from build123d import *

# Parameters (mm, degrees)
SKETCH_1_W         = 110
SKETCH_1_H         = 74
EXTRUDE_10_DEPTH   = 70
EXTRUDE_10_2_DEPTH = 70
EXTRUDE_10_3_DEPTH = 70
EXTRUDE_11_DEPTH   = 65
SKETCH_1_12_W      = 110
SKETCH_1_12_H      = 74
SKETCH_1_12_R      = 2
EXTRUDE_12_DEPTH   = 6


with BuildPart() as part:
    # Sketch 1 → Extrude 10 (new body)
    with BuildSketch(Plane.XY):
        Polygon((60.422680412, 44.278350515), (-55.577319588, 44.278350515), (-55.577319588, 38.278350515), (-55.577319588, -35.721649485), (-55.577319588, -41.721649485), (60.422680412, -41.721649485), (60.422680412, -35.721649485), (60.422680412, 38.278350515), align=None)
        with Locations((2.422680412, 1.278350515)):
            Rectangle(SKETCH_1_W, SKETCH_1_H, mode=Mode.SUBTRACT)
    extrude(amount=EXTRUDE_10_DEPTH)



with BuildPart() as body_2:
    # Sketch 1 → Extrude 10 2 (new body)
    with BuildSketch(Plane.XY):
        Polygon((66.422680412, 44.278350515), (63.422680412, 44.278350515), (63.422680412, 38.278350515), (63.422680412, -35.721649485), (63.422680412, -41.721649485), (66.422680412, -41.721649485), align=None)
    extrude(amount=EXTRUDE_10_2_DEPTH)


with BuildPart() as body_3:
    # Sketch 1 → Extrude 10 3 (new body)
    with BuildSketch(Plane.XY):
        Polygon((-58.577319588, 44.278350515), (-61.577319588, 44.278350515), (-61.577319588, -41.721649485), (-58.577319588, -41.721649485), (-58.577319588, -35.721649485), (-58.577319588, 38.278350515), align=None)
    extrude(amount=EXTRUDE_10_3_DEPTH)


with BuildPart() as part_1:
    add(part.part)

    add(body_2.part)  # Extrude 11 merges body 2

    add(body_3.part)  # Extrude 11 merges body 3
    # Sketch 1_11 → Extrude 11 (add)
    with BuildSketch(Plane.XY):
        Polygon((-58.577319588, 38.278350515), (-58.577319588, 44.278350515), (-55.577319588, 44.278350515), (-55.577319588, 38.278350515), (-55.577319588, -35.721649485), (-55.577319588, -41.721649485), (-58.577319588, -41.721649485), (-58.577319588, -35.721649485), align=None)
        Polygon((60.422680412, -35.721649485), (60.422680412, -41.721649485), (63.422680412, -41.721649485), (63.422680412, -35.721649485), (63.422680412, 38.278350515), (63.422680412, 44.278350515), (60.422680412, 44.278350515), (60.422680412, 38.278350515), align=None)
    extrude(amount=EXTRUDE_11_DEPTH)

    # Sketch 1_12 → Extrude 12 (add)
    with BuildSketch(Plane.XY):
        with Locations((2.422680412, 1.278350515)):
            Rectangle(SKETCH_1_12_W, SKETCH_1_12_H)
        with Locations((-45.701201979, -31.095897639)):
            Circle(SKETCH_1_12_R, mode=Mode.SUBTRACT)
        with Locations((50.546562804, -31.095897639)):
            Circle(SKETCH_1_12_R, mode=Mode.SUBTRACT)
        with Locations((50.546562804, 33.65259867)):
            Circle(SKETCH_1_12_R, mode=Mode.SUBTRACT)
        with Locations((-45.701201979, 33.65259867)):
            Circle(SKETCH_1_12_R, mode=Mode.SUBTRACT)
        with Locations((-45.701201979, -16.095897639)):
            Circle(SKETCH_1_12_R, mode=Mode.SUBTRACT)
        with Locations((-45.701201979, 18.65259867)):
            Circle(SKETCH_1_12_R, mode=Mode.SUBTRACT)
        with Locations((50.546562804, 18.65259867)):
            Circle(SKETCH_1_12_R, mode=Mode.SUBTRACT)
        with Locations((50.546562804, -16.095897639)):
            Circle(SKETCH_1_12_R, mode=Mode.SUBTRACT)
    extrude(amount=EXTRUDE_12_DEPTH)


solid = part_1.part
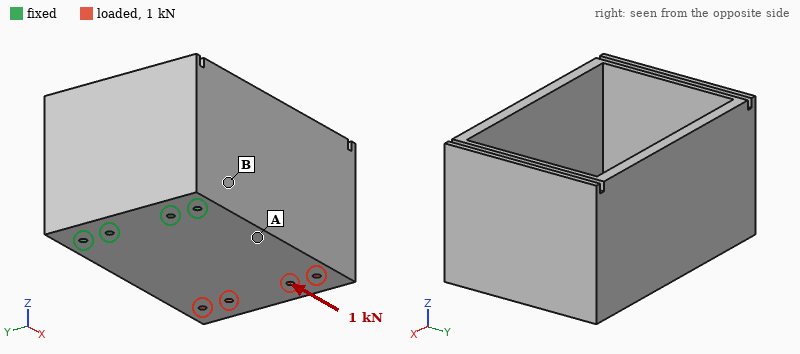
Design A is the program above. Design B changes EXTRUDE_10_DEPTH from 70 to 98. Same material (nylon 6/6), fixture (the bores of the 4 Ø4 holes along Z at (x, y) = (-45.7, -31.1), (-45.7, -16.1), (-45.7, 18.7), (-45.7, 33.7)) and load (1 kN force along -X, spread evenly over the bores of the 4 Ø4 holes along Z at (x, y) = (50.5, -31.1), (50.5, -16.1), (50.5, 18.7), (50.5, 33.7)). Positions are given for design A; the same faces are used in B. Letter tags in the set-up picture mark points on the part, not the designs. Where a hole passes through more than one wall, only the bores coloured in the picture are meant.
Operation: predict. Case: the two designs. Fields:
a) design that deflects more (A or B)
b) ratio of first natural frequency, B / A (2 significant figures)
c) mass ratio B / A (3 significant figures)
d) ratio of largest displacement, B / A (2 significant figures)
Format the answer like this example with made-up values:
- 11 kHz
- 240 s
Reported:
- A
- 0.85
- 1.21
- 0.89
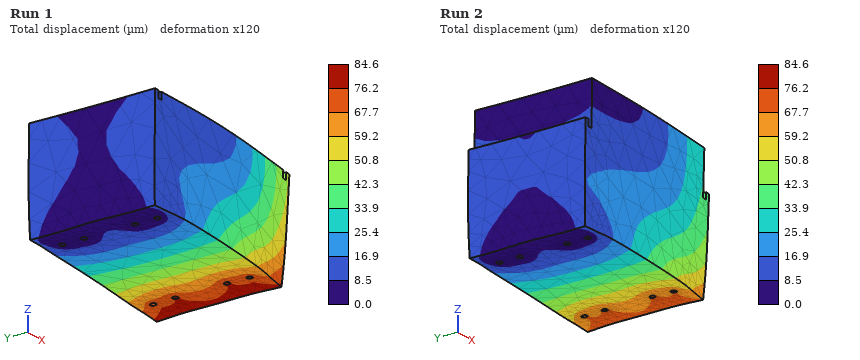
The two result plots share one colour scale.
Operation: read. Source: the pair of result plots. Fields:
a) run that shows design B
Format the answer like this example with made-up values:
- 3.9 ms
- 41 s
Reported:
- Run 2
